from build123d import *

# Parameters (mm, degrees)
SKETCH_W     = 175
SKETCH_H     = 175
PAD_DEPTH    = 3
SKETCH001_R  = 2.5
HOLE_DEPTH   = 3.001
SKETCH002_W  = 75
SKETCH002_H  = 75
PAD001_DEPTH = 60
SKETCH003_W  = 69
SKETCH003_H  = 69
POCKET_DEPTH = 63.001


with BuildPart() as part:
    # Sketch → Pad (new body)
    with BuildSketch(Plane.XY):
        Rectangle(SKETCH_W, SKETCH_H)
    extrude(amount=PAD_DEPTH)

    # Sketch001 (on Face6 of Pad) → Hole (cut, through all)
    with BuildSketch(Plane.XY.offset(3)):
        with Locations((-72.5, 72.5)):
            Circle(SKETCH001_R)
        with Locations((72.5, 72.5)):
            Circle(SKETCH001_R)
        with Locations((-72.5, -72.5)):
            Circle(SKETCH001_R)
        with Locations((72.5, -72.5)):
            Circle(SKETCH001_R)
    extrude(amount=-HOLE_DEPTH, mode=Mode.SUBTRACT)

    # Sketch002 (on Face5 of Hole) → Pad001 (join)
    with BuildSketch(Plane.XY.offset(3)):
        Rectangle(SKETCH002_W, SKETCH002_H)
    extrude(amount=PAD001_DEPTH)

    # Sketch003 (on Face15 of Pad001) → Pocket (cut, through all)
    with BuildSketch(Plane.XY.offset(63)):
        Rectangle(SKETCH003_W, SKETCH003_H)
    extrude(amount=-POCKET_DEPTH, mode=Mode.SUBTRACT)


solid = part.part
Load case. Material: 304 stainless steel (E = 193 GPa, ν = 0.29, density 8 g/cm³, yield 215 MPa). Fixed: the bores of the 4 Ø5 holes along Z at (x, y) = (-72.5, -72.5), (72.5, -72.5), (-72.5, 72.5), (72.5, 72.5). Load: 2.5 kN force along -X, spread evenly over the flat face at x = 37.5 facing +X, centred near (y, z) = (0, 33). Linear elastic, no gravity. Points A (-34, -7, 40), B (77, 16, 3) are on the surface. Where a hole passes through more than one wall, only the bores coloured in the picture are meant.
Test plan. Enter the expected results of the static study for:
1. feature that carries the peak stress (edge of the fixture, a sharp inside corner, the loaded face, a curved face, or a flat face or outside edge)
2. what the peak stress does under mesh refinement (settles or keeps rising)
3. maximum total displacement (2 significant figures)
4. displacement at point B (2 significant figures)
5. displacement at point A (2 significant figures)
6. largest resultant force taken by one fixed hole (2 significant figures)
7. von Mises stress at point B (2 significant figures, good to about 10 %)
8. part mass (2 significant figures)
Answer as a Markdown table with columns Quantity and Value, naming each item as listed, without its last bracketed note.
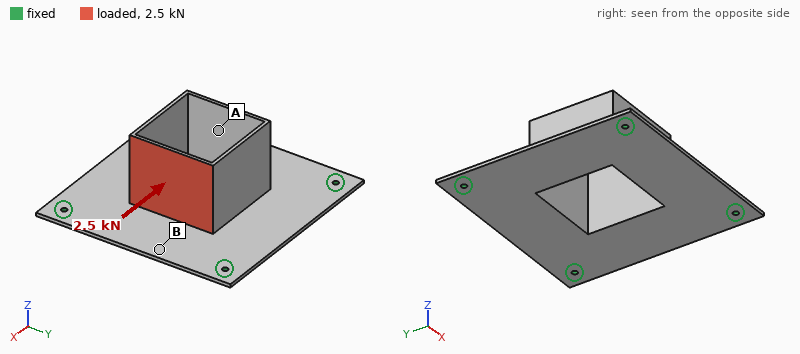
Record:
| Quantity | Value |
|---|---|
| feature that carries the peak stress | edge of the fixture |
| what the peak stress does under mesh refinement | keeps rising |
| maximum total displacement | 0.42 mm |
| displacement at point B | 0.19 mm |
| displacement at point A | 0.17 mm |
| largest resultant force taken by one fixed hole | 790 N |
| von Mises stress at point B | 35 MPa |
| part mass | 1.0 kg |
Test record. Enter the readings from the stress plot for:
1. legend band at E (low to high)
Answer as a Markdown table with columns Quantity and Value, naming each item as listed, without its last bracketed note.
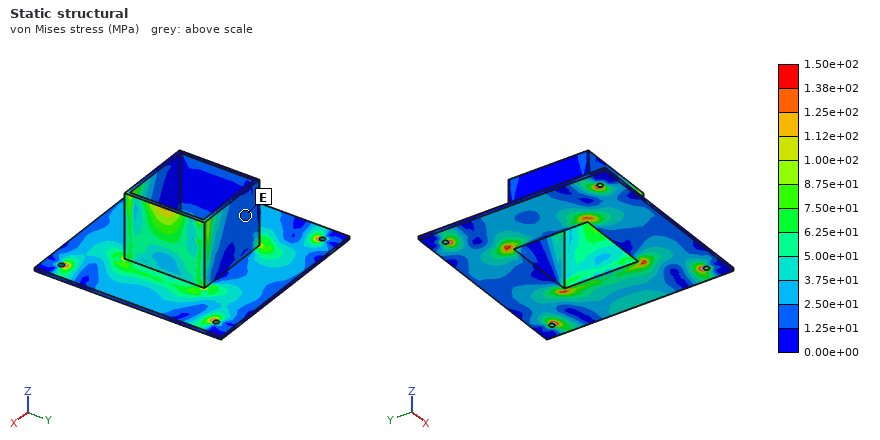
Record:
| Quantity | Value |
|---|---|
| legend band at E | 1.25e+01 to 2.50e+01 MPa |
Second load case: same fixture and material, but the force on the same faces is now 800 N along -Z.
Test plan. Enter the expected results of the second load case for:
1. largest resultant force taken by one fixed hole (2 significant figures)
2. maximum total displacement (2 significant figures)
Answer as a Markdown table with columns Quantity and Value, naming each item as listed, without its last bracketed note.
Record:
| Quantity | Value |
|---|---|
| largest resultant force taken by one fixed hole | 360 N |
| maximum total displacement | 0.20 mm |
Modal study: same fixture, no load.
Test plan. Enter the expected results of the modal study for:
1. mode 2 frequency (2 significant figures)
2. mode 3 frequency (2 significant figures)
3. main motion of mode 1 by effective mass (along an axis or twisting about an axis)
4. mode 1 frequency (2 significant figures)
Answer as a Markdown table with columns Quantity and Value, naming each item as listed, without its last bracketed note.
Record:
| Quantity | Value |
|---|---|
| mode 2 frequency | 630 Hz |
| mode 3 frequency | 630 Hz |
| main motion of mode 1 by effective mass | along Z |
| mode 1 frequency | 470 Hz |
